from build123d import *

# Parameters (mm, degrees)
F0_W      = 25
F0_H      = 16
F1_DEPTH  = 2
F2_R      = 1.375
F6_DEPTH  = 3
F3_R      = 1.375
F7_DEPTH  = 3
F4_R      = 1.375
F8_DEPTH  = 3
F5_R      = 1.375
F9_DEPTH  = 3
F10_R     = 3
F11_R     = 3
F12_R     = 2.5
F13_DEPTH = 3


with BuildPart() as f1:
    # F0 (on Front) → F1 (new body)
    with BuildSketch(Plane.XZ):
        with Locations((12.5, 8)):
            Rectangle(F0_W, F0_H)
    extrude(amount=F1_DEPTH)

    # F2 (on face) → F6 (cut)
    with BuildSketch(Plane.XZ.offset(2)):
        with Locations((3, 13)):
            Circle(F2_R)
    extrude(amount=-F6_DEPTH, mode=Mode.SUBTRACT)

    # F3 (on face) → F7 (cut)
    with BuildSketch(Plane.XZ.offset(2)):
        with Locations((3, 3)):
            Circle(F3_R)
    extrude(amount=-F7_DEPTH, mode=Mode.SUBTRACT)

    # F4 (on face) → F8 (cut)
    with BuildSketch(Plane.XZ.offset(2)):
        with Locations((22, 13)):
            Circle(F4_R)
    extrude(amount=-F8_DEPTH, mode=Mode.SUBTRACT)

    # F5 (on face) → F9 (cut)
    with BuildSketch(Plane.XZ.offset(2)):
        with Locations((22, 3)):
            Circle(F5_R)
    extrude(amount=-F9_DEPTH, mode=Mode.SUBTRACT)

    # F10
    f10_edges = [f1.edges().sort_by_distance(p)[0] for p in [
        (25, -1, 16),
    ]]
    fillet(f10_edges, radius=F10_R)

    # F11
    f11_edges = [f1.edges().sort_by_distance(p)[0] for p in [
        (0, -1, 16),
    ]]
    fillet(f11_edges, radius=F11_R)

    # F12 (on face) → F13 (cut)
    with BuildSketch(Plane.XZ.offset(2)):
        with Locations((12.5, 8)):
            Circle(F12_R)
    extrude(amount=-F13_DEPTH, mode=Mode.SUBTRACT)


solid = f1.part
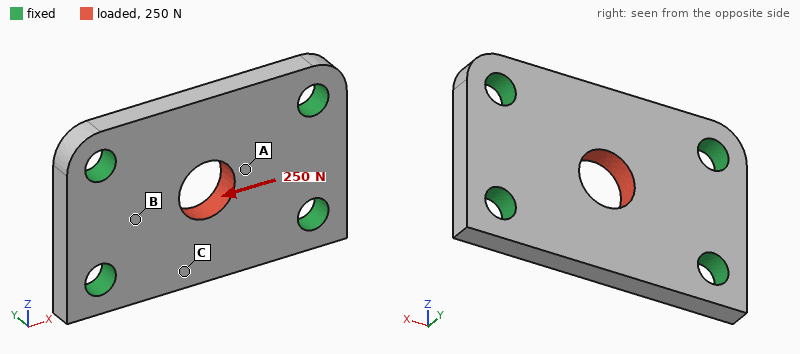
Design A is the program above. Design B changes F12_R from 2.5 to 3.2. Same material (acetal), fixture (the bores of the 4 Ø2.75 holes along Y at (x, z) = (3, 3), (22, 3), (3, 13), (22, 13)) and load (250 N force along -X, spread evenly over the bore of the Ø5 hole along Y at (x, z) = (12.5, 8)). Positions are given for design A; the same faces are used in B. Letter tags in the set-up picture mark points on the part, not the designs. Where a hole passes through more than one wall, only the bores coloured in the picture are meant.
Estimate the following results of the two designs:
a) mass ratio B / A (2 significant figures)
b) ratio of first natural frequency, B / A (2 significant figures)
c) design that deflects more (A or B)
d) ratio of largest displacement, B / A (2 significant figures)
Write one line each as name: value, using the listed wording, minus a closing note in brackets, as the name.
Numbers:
mass ratio B / A: 0.96
ratio of first natural frequency, B / A: 1.0
design that deflects more: A
ratio of largest displacement, B / A: 0.87
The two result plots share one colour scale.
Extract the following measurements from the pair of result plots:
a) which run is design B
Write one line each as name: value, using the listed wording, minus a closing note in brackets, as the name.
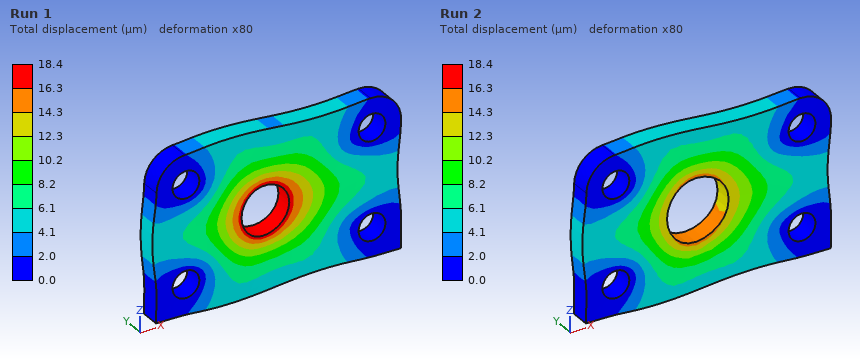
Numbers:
which run is design B: Run 2
